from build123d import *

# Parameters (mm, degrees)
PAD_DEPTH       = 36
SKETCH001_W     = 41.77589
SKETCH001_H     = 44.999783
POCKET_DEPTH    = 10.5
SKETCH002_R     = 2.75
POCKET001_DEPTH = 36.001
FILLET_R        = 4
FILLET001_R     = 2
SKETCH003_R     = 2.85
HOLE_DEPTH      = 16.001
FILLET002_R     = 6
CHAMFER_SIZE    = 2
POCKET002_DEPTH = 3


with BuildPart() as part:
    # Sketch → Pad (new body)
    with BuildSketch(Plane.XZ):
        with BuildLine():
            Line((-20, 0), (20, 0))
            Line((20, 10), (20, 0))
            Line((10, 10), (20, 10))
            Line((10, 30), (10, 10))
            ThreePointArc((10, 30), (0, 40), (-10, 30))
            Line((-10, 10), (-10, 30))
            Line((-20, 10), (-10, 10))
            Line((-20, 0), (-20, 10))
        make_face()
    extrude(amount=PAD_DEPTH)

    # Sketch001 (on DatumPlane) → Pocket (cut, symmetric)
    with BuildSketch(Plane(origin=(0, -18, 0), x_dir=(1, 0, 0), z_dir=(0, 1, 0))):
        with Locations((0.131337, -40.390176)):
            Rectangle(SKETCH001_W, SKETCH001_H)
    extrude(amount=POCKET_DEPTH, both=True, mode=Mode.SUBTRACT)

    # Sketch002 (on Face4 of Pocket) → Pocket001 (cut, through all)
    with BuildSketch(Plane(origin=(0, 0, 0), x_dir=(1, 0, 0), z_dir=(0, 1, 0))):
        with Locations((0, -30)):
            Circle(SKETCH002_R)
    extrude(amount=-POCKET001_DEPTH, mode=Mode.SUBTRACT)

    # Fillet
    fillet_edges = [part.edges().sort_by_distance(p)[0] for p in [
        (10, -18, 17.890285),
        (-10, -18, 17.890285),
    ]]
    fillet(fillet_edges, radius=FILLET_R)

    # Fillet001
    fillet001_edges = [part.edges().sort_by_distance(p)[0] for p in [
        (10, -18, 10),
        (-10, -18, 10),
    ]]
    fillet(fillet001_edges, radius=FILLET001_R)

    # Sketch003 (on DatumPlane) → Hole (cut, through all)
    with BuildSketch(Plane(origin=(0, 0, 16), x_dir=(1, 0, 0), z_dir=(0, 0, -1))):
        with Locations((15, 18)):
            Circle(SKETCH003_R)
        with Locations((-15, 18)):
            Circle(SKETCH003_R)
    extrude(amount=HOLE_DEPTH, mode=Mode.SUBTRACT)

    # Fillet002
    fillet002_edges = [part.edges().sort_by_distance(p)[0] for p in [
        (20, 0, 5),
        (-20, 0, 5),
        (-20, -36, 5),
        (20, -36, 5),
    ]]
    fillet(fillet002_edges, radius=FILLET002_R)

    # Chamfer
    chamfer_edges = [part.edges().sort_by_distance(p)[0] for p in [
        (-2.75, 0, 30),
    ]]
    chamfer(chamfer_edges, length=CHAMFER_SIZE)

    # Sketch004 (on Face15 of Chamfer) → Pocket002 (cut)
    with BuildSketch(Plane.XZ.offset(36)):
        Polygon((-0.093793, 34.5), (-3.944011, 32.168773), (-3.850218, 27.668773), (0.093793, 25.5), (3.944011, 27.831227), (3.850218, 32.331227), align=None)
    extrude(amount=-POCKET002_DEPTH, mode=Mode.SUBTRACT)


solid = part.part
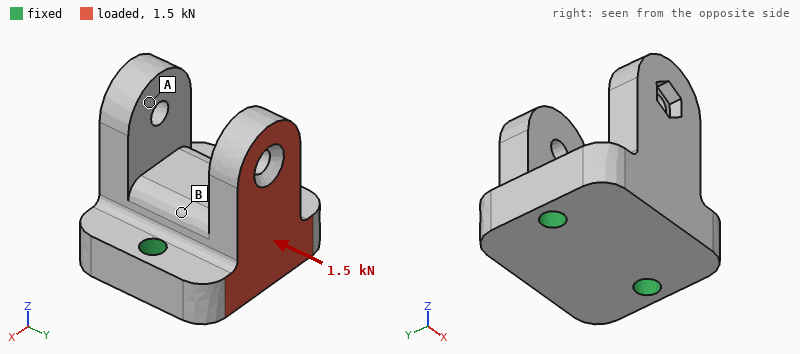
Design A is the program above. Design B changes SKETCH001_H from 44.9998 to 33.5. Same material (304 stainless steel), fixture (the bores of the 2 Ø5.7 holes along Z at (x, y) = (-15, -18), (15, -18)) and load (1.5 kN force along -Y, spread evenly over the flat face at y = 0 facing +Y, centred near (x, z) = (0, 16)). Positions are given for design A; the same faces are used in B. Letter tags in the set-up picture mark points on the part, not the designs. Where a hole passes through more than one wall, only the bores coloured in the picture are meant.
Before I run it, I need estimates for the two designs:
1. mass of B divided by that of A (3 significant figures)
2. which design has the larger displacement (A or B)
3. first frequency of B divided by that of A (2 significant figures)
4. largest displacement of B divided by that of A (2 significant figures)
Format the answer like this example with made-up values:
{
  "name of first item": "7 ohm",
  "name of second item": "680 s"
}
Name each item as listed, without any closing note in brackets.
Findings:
{
  "mass of B divided by that of A": "1.10",
  "which design has the larger displacement": "A",
  "first frequency of B divided by that of A": "1.1",
  "largest displacement of B divided by that of A": "0.58"
}
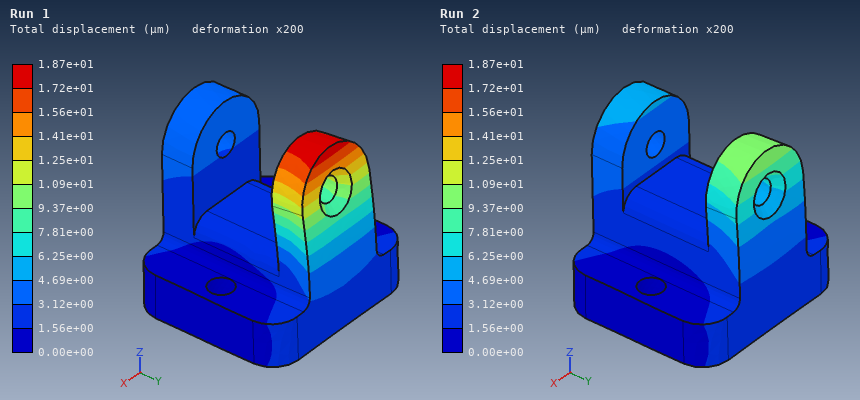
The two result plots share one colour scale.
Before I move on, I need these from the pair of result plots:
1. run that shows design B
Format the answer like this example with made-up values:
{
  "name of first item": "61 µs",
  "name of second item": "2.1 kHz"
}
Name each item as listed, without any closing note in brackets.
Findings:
{
  "run that shows design B": "Run 2"
}
